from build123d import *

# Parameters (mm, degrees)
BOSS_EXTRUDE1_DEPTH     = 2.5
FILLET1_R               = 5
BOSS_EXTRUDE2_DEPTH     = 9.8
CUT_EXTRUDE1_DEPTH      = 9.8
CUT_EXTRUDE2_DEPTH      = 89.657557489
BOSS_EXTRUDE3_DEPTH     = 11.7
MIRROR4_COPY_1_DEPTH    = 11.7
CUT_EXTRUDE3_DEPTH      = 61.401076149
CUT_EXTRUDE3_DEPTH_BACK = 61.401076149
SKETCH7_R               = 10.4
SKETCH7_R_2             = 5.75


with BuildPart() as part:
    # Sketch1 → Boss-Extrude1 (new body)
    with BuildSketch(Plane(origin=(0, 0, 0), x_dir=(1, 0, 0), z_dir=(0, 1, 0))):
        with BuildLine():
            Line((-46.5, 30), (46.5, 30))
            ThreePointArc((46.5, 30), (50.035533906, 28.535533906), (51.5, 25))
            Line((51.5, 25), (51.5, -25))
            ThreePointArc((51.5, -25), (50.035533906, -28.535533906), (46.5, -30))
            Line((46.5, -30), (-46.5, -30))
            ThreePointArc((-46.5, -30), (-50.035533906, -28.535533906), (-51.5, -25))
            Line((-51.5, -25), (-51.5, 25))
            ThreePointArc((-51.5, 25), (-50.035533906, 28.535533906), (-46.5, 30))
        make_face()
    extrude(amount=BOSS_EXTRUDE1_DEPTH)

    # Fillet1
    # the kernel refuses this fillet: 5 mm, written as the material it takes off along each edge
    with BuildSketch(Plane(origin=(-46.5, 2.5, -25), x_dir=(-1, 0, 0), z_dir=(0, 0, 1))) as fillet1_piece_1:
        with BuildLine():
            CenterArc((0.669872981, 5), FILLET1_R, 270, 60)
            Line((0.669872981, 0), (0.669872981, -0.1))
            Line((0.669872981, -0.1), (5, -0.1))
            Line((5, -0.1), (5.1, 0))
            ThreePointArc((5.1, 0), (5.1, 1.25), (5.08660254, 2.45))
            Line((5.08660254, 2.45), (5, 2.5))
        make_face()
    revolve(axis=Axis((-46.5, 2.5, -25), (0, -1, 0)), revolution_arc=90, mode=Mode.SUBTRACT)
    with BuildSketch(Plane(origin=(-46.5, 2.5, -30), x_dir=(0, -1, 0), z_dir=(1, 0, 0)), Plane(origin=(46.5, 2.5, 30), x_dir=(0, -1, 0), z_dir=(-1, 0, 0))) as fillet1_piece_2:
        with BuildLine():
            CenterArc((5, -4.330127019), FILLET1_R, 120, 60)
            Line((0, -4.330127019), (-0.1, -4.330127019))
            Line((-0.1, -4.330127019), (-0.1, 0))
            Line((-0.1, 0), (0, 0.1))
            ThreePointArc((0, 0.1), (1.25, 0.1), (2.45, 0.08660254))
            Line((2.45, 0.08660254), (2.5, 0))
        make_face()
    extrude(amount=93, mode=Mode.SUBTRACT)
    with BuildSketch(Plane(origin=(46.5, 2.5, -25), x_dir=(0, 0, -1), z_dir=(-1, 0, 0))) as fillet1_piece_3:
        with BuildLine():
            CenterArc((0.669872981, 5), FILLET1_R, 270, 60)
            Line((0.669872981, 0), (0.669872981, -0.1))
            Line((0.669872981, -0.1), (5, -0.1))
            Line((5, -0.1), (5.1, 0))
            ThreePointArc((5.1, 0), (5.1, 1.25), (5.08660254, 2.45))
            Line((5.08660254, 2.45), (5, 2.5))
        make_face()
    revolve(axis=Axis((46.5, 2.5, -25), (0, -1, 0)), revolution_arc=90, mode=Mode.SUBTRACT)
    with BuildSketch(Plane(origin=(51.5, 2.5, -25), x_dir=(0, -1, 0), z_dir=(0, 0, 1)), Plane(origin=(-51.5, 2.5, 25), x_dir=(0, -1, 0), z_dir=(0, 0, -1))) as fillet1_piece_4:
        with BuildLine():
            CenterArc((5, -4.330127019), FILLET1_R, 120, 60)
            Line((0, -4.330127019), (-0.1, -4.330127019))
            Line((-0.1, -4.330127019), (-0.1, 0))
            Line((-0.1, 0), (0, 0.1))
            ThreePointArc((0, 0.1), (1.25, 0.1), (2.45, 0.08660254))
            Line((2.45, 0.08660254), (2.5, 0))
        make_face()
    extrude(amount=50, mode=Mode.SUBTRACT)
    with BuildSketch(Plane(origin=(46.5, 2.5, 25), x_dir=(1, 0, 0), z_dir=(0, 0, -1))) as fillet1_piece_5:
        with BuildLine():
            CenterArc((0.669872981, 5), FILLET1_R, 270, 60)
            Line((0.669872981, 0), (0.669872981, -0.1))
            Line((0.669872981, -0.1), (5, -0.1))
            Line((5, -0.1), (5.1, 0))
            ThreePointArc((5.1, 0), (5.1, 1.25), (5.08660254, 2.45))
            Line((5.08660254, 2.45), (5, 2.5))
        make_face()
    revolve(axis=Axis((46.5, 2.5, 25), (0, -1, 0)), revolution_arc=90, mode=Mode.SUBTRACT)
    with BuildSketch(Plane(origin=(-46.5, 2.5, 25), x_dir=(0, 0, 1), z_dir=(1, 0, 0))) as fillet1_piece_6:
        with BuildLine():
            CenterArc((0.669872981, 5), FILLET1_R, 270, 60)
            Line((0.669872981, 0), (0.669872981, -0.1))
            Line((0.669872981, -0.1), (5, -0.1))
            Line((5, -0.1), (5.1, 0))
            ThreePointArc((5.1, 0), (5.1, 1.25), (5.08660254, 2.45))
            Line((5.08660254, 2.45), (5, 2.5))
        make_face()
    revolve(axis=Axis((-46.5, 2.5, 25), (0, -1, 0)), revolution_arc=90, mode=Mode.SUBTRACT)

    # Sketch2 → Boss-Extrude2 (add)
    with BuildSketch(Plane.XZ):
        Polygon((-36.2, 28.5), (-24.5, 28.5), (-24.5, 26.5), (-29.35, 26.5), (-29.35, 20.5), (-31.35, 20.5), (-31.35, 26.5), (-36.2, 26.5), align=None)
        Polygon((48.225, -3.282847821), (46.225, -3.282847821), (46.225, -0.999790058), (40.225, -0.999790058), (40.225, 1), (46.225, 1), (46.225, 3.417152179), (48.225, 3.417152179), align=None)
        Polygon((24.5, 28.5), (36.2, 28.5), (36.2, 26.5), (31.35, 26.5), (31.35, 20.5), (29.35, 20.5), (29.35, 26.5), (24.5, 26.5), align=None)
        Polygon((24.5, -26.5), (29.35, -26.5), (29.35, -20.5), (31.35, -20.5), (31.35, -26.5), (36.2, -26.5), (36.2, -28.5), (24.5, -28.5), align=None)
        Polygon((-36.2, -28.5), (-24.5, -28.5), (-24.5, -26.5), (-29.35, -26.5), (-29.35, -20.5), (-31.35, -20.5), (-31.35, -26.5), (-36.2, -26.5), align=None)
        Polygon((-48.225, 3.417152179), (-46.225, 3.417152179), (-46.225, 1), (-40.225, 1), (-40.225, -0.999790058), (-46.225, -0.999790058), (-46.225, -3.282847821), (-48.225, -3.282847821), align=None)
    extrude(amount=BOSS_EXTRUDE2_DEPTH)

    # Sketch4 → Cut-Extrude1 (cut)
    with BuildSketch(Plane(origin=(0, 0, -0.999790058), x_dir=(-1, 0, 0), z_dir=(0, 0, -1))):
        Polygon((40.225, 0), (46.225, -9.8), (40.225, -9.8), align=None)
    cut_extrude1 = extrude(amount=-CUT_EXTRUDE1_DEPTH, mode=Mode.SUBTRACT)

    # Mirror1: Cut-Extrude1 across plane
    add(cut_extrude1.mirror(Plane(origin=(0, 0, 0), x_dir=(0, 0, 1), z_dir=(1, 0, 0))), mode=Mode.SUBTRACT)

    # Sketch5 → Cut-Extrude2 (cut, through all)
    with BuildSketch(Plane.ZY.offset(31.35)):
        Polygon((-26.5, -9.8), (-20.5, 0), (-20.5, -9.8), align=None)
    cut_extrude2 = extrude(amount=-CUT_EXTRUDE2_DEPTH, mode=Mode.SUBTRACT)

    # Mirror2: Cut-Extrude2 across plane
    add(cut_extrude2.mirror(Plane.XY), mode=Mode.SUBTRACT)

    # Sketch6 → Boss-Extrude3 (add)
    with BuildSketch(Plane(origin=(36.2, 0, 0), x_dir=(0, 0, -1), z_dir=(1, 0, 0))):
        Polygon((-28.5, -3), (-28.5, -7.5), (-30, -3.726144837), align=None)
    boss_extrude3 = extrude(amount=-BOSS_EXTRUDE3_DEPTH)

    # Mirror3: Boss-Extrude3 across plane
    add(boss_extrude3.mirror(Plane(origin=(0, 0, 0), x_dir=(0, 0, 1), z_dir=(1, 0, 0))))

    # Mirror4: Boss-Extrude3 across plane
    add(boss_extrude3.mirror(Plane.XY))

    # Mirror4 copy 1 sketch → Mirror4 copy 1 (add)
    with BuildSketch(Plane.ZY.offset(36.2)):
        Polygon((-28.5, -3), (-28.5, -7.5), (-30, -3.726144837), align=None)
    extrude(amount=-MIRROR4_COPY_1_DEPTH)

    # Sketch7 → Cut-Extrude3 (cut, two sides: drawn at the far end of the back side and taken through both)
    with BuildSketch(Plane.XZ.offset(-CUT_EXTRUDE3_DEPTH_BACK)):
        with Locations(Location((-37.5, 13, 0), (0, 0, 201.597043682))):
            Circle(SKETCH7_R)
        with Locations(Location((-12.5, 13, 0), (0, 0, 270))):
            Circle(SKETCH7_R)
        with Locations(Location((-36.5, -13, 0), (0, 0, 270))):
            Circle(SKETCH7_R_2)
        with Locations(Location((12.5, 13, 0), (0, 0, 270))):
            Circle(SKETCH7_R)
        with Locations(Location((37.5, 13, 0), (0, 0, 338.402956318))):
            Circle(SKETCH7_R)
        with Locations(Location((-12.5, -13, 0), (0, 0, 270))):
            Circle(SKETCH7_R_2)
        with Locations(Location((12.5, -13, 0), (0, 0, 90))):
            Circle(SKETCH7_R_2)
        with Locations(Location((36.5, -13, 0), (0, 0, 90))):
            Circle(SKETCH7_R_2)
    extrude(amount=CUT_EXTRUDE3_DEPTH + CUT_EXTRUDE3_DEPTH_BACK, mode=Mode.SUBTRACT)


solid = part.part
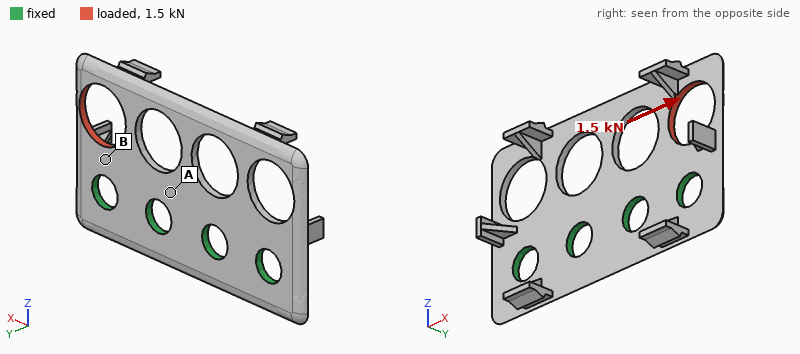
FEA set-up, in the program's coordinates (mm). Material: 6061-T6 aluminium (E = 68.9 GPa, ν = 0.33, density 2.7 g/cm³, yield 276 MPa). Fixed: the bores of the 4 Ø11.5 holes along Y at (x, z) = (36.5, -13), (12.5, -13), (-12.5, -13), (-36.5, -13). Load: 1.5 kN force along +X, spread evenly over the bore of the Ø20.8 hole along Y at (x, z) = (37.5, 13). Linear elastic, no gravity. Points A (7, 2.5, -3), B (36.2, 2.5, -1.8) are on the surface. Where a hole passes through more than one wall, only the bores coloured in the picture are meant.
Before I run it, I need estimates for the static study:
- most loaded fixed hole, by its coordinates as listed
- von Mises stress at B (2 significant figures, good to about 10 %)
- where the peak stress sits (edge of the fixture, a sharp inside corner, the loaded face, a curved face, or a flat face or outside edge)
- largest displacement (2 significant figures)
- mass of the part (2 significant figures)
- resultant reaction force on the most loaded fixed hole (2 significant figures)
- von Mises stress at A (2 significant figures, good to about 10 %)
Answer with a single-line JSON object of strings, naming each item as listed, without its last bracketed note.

{"most loaded fixed hole, by its coordinates as listed": "(36.5, -13)", "von Mises stress at B": "38 MPa", "where the peak stress sits": "the loaded face", "largest displacement": "67 µm", "mass of the part": "32 g", "resultant reaction force on the most loaded fixed hole": "870 N", "von Mises stress at A": "16 MPa"}
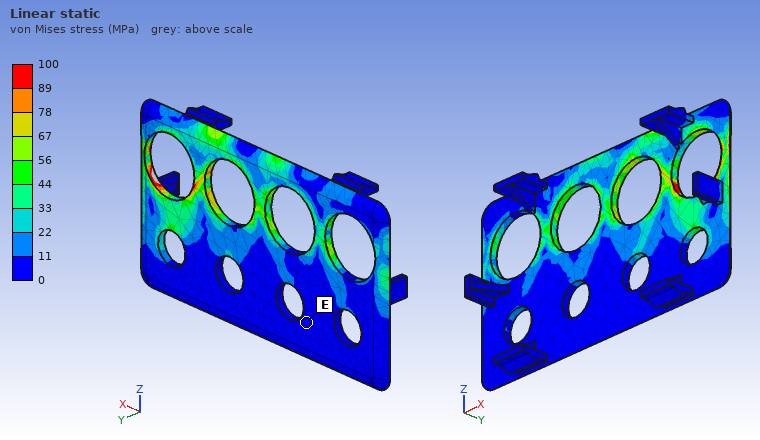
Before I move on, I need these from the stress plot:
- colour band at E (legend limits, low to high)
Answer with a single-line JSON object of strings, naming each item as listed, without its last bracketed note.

{"colour band at E": "0 to 11 MPa"}
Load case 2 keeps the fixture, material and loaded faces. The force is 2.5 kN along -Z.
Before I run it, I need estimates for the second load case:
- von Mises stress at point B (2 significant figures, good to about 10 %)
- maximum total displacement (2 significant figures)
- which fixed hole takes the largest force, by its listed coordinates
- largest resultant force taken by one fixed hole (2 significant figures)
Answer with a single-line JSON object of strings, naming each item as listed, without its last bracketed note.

{"von Mises stress at point B": "31 MPa", "maximum total displacement": "75 µm", "which fixed hole takes the largest force, by its listed coordinates": "(36.5, -13)", "largest resultant force taken by one fixed hole": "2.1 kN"}
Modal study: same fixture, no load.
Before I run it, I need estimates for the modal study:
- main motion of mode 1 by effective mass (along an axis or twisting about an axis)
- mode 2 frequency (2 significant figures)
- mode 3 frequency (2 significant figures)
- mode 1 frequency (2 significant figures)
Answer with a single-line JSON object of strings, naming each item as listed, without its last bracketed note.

{"main motion of mode 1 by effective mass": "along Y", "mode 2 frequency": "1400 Hz", "mode 3 frequency": "2600 Hz", "mode 1 frequency": "1100 Hz"}
